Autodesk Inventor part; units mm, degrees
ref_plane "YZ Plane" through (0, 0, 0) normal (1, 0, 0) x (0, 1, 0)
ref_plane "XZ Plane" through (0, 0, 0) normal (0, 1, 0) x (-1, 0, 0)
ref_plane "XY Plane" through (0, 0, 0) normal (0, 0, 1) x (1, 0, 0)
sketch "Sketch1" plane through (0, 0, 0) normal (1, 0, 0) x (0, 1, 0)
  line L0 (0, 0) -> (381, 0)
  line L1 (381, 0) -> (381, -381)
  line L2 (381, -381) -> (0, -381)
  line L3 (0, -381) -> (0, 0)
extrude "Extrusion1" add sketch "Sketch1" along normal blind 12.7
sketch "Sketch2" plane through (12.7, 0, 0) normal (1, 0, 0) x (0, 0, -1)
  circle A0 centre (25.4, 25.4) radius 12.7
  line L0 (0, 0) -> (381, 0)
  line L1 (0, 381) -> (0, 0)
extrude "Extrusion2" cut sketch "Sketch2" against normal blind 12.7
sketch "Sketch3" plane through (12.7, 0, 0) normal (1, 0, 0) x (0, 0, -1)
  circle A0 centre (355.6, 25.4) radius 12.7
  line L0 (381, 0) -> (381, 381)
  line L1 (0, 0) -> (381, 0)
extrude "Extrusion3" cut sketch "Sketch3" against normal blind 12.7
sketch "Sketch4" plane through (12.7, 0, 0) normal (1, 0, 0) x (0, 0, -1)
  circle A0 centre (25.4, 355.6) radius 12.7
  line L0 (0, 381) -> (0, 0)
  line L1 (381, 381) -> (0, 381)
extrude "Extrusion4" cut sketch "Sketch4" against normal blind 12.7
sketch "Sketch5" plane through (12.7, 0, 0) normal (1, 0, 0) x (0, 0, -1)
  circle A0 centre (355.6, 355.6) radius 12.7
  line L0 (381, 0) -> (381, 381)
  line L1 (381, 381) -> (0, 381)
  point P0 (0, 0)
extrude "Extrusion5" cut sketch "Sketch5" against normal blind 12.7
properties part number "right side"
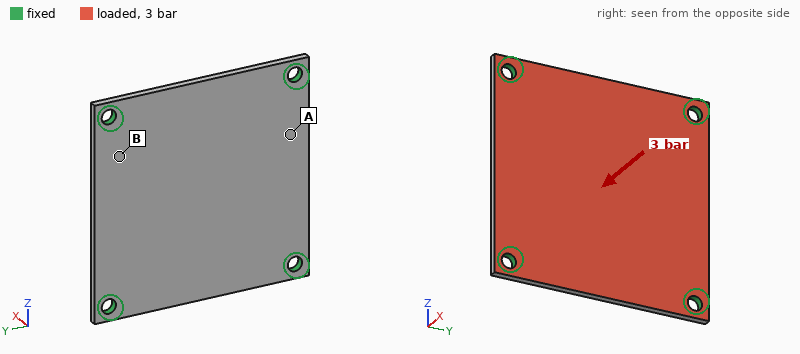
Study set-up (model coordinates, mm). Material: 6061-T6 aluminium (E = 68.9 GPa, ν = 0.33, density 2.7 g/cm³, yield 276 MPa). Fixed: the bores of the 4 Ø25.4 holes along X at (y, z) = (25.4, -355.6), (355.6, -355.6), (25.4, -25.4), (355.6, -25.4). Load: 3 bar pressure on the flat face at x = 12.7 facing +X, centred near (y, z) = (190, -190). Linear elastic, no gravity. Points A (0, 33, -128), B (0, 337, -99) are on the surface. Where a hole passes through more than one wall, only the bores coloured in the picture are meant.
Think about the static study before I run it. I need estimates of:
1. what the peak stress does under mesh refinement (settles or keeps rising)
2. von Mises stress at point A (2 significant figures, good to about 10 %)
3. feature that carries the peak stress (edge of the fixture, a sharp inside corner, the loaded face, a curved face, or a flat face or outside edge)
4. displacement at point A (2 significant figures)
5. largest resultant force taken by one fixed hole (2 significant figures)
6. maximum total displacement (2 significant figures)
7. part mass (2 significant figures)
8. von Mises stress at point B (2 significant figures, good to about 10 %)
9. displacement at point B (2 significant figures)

keeps rising
40 MPa
edge of the fixture
0.78 mm
11 kN
1.9 mm
4.9 kg
24 MPa
0.60 mm
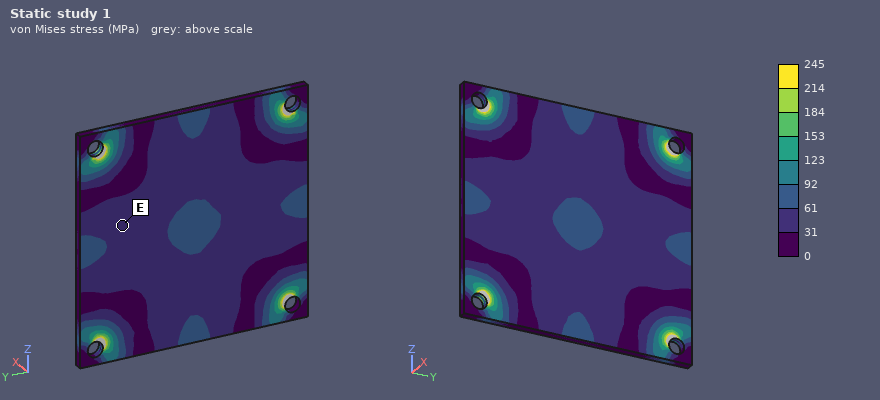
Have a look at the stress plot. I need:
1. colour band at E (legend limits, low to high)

31 to 61 MPa
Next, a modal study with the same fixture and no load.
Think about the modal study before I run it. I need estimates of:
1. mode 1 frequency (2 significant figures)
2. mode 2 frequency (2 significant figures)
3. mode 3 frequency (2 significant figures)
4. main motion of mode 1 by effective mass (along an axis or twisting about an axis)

420 Hz
710 Hz
710 Hz
along X
